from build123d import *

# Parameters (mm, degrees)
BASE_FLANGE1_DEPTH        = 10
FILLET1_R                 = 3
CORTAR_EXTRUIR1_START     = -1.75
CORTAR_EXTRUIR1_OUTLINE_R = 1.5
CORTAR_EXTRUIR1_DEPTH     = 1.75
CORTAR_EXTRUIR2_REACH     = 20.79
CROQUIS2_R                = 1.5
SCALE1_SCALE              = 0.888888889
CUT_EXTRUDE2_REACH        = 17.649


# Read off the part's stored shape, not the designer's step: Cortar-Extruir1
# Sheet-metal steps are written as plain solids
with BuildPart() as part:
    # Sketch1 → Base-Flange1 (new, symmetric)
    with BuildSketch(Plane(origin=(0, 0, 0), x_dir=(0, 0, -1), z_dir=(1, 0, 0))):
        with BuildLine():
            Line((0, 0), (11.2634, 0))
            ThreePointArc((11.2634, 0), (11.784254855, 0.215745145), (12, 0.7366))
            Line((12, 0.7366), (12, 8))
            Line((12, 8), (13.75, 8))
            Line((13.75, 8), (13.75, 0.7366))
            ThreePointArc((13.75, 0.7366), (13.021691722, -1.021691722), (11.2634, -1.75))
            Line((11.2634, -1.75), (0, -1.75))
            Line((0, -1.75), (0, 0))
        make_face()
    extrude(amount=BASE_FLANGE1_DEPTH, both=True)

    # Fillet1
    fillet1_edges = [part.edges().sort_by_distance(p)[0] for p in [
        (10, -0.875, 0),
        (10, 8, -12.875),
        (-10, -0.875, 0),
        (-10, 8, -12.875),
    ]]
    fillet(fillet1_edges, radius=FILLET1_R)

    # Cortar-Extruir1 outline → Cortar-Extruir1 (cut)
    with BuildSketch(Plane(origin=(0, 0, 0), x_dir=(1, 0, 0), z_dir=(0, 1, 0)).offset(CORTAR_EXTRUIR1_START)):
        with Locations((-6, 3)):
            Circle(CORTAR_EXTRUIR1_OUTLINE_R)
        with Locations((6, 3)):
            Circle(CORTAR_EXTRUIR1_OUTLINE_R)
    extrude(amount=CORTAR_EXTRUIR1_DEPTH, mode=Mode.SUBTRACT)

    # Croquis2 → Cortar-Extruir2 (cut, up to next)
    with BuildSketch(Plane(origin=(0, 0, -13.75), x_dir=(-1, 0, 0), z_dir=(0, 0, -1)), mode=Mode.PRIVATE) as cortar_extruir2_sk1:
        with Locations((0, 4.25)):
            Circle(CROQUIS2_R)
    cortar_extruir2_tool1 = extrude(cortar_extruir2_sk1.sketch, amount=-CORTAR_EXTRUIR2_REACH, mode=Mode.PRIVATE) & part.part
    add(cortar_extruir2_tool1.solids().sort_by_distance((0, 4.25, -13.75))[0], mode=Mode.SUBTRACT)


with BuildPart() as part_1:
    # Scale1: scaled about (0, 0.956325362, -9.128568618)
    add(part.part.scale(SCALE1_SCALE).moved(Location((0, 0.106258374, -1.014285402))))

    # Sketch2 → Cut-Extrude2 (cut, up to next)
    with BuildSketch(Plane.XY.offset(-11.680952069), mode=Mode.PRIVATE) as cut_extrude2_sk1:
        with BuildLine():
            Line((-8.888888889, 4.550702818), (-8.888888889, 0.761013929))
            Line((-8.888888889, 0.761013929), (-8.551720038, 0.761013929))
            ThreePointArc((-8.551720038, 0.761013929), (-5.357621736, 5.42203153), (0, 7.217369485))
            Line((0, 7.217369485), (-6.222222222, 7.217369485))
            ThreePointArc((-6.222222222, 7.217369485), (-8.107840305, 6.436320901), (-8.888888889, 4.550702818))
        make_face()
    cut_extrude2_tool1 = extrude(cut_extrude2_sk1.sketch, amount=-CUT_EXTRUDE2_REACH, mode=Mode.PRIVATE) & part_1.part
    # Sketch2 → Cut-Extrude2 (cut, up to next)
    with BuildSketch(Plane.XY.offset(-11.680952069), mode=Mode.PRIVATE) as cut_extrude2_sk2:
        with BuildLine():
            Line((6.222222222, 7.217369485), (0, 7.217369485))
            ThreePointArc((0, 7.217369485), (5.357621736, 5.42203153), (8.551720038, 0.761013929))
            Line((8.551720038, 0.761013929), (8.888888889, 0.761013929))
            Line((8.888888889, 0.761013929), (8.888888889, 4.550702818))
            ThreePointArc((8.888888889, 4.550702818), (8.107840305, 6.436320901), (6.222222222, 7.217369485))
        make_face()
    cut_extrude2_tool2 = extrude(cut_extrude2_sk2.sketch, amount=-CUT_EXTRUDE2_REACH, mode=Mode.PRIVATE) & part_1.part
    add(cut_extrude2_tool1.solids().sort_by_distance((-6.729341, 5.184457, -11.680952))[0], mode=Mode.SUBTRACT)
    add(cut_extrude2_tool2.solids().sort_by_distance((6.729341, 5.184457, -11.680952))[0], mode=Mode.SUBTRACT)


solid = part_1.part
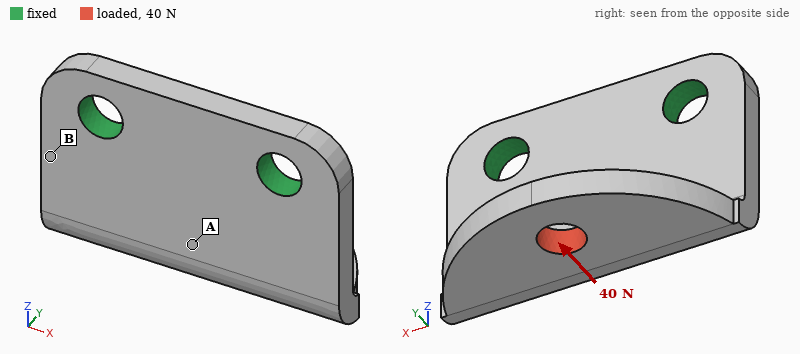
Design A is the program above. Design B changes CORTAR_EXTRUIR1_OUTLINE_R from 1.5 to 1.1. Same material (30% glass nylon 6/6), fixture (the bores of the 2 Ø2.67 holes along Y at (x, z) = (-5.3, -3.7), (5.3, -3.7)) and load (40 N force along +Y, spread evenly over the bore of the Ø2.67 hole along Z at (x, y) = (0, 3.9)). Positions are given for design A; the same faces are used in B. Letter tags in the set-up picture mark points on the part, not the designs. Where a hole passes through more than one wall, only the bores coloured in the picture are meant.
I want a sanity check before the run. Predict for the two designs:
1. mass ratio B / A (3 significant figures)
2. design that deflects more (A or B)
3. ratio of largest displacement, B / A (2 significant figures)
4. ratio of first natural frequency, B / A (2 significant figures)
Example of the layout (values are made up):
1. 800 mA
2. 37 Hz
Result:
1. 1.02
2. B
3. 1.2
4. 0.93
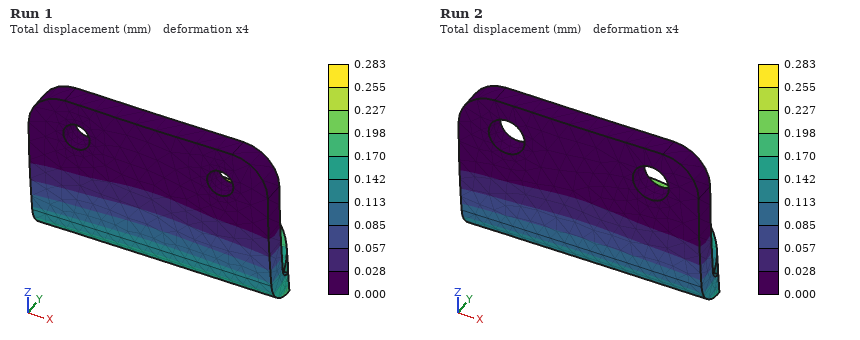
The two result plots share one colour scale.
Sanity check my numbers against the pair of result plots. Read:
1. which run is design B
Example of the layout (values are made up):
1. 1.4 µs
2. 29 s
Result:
1. Run 1
